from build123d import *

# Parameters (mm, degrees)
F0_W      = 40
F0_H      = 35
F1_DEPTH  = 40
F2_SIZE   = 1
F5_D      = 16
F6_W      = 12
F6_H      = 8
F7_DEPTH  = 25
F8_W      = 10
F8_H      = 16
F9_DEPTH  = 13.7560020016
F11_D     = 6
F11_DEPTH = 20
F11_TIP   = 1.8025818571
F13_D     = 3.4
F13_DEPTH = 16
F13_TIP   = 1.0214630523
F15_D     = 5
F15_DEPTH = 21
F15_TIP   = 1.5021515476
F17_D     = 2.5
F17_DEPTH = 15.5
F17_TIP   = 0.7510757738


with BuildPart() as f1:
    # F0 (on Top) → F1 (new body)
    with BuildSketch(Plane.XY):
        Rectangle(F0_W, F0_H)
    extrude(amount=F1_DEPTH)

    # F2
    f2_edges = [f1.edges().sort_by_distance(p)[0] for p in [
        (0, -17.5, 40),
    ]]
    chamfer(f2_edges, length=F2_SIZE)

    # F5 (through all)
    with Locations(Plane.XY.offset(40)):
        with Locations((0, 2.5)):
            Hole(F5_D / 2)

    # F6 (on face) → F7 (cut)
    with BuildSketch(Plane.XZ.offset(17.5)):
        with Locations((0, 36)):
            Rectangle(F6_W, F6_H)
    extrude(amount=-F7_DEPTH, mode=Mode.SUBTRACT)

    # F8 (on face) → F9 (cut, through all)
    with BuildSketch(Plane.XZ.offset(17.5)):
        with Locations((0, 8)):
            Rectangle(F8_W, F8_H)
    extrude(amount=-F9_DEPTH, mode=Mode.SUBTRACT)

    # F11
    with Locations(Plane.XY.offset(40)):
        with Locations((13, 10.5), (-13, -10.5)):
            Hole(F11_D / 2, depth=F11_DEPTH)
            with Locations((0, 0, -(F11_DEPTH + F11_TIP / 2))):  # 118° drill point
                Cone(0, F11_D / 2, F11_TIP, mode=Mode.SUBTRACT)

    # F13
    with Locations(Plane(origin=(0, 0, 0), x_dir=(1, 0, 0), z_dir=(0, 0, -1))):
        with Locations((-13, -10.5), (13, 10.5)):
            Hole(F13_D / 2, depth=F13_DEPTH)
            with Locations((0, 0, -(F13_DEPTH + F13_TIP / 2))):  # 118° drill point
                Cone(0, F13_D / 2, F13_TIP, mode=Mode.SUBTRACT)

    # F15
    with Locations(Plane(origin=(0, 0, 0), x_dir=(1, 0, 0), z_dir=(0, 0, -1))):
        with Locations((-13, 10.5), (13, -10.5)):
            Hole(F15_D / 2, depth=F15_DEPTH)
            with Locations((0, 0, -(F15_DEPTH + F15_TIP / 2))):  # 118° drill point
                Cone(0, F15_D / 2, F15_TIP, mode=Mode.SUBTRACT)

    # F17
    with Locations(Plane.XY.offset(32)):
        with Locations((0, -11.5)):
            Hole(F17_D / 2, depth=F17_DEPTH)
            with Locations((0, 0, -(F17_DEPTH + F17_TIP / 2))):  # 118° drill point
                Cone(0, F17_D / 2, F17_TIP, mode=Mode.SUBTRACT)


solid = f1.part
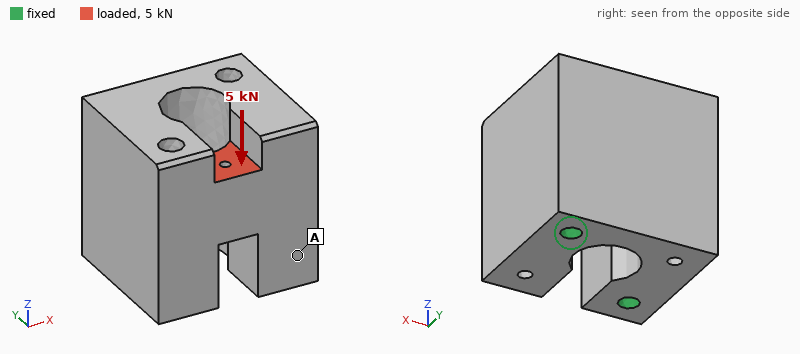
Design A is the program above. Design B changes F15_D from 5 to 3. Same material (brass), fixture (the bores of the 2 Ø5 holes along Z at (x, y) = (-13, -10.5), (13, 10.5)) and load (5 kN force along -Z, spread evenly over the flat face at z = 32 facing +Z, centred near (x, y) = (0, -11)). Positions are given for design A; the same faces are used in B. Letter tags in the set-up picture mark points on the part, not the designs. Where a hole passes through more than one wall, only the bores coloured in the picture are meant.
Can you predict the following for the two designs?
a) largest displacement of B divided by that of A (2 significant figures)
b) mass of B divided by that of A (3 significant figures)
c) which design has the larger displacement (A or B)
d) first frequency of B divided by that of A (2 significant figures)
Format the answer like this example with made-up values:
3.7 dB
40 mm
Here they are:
1.2
1.01
B
0.85
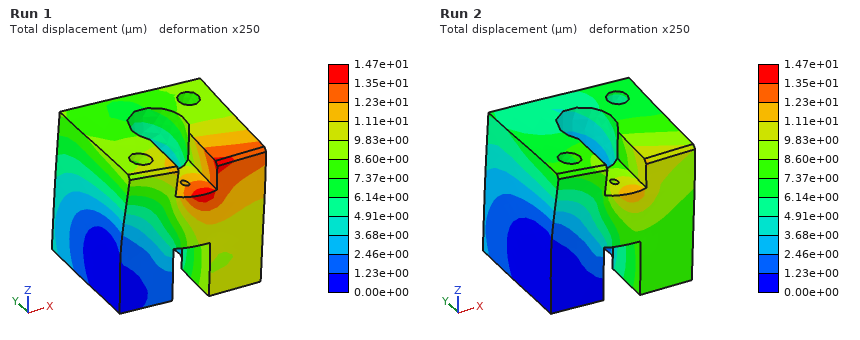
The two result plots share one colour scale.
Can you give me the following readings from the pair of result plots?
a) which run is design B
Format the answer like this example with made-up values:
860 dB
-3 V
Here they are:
Run 1
